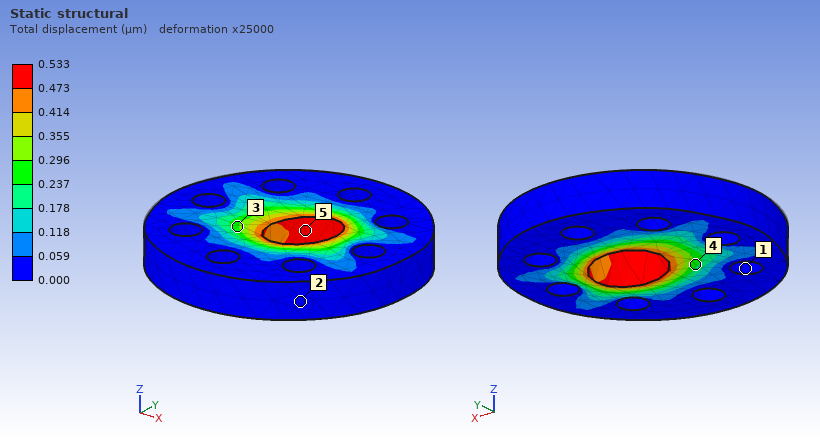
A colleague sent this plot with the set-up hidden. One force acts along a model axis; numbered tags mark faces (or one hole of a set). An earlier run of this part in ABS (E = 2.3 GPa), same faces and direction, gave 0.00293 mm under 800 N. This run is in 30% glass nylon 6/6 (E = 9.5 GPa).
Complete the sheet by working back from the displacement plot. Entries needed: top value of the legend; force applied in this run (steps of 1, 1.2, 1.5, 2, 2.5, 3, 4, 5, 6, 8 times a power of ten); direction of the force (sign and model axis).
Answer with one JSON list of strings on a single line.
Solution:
["0.533 µm", "600 N", "+X"]
